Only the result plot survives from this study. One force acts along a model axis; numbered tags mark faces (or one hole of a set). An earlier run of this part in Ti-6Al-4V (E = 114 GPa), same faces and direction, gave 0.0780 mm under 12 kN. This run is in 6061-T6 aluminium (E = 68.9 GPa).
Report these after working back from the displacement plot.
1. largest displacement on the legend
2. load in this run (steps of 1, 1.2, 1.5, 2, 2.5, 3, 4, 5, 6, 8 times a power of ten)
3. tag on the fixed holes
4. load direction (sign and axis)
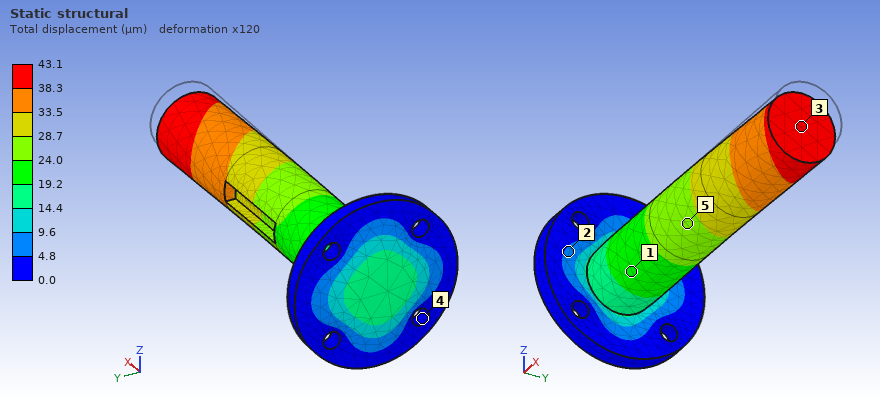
43.1 µm
4 kN
4
-X
